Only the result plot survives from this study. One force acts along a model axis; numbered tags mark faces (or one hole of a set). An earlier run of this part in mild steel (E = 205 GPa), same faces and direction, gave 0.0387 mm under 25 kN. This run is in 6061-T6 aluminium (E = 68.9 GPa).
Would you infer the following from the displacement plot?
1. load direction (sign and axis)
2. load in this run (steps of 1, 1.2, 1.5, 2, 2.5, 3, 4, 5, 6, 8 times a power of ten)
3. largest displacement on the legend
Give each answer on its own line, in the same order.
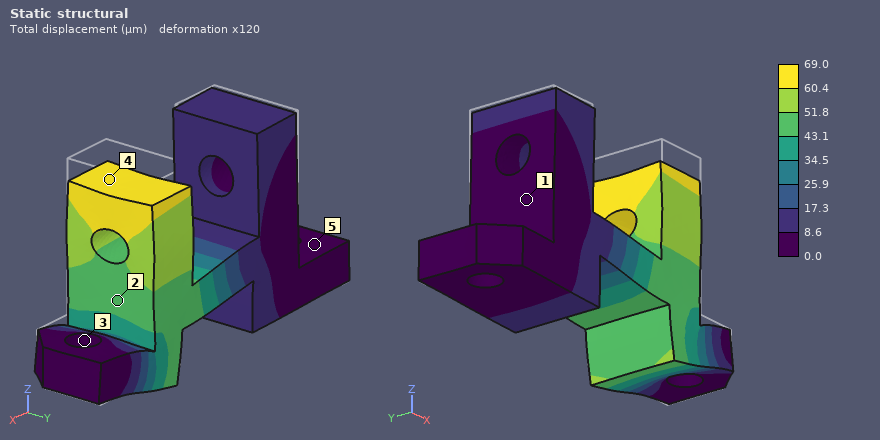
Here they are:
-Z
15 kN
69.0 µm
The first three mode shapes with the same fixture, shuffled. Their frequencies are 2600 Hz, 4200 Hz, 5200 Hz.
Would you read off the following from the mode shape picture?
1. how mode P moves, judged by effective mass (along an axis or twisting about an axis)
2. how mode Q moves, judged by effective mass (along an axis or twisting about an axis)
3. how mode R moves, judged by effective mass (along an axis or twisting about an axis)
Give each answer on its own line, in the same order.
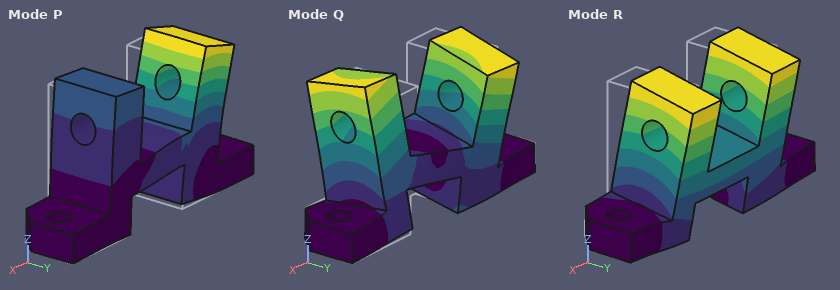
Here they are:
along X
twisting about Z
along Y
